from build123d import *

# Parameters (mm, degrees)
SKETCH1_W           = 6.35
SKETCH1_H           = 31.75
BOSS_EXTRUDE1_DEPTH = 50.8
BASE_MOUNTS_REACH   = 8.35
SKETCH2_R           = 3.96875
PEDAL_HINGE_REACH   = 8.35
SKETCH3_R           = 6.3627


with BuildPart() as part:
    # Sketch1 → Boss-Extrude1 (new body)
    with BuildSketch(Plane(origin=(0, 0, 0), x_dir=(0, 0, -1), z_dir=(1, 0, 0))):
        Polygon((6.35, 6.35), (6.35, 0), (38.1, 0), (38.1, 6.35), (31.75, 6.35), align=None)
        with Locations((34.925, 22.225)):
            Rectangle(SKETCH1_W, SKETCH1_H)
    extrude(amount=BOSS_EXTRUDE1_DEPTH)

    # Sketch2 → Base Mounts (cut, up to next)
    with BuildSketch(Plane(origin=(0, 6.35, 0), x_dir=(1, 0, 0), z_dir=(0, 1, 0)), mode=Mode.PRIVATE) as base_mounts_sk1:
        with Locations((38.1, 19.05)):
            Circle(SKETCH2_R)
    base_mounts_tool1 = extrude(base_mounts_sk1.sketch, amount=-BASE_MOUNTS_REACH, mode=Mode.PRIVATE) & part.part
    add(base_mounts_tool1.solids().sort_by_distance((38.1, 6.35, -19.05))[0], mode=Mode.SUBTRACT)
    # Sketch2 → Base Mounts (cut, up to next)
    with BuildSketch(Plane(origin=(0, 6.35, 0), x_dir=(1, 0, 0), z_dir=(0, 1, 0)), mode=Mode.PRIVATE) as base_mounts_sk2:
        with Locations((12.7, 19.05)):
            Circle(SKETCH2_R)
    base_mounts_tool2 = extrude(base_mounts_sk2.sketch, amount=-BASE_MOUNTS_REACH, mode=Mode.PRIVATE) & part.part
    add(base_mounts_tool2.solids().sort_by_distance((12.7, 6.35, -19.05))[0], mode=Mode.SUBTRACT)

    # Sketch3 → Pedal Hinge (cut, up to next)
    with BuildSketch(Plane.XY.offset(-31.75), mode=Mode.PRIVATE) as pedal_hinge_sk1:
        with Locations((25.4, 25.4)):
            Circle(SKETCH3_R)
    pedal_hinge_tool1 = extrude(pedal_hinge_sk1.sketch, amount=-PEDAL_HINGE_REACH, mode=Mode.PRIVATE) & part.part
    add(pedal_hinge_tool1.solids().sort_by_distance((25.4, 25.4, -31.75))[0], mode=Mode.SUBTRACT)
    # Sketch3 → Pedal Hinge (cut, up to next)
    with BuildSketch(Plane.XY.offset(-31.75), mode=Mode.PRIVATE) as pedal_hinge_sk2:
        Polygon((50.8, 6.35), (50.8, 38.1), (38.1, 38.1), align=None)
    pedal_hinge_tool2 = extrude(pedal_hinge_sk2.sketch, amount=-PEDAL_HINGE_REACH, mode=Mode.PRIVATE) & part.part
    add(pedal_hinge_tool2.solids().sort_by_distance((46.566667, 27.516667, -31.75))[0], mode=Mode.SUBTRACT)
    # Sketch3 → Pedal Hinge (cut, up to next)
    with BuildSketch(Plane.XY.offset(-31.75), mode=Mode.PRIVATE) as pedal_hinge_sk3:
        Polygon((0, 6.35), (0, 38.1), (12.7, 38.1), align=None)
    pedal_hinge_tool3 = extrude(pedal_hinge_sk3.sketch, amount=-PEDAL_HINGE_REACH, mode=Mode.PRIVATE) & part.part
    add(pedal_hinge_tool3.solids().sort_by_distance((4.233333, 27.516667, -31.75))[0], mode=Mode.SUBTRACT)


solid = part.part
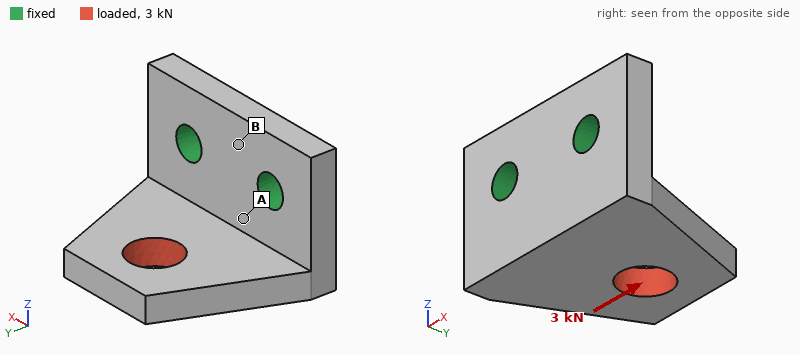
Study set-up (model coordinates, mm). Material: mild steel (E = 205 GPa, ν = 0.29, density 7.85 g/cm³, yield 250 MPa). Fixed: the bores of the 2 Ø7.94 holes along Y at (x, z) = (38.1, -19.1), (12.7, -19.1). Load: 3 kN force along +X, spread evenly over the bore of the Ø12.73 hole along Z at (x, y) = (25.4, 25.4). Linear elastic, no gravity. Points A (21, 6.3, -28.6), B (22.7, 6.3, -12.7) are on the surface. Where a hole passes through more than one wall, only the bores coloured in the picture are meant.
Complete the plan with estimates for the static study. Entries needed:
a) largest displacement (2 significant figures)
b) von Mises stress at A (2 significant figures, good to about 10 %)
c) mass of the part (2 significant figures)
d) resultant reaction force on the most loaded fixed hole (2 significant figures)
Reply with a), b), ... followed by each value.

a) 40 µm
b) 78 MPa
c) 130 g
d) 2.9 kN
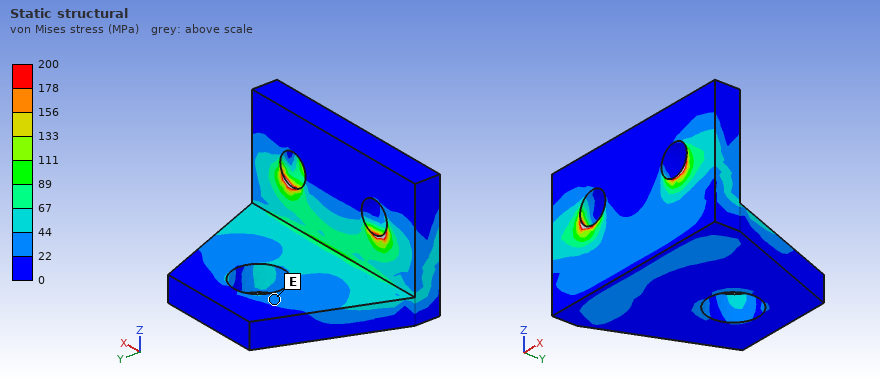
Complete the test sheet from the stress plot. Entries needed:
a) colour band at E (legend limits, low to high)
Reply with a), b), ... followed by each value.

a) 22 to 44 MPa
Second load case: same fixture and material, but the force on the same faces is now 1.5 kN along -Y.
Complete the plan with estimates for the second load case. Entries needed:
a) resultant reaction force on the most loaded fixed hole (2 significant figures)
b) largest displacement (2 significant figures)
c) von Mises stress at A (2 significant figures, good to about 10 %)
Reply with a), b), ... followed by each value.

a) 750 N
b) 27 µm
c) 24 MPa
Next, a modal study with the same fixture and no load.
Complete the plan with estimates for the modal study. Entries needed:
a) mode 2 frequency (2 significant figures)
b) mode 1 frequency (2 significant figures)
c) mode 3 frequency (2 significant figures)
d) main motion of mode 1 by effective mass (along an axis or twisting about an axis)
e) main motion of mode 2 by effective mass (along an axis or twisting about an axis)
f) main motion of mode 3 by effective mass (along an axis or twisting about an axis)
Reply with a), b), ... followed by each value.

a) 7200 Hz
b) 3500 Hz
c) 11 kHz
d) along Z
e) along X
f) along Y
